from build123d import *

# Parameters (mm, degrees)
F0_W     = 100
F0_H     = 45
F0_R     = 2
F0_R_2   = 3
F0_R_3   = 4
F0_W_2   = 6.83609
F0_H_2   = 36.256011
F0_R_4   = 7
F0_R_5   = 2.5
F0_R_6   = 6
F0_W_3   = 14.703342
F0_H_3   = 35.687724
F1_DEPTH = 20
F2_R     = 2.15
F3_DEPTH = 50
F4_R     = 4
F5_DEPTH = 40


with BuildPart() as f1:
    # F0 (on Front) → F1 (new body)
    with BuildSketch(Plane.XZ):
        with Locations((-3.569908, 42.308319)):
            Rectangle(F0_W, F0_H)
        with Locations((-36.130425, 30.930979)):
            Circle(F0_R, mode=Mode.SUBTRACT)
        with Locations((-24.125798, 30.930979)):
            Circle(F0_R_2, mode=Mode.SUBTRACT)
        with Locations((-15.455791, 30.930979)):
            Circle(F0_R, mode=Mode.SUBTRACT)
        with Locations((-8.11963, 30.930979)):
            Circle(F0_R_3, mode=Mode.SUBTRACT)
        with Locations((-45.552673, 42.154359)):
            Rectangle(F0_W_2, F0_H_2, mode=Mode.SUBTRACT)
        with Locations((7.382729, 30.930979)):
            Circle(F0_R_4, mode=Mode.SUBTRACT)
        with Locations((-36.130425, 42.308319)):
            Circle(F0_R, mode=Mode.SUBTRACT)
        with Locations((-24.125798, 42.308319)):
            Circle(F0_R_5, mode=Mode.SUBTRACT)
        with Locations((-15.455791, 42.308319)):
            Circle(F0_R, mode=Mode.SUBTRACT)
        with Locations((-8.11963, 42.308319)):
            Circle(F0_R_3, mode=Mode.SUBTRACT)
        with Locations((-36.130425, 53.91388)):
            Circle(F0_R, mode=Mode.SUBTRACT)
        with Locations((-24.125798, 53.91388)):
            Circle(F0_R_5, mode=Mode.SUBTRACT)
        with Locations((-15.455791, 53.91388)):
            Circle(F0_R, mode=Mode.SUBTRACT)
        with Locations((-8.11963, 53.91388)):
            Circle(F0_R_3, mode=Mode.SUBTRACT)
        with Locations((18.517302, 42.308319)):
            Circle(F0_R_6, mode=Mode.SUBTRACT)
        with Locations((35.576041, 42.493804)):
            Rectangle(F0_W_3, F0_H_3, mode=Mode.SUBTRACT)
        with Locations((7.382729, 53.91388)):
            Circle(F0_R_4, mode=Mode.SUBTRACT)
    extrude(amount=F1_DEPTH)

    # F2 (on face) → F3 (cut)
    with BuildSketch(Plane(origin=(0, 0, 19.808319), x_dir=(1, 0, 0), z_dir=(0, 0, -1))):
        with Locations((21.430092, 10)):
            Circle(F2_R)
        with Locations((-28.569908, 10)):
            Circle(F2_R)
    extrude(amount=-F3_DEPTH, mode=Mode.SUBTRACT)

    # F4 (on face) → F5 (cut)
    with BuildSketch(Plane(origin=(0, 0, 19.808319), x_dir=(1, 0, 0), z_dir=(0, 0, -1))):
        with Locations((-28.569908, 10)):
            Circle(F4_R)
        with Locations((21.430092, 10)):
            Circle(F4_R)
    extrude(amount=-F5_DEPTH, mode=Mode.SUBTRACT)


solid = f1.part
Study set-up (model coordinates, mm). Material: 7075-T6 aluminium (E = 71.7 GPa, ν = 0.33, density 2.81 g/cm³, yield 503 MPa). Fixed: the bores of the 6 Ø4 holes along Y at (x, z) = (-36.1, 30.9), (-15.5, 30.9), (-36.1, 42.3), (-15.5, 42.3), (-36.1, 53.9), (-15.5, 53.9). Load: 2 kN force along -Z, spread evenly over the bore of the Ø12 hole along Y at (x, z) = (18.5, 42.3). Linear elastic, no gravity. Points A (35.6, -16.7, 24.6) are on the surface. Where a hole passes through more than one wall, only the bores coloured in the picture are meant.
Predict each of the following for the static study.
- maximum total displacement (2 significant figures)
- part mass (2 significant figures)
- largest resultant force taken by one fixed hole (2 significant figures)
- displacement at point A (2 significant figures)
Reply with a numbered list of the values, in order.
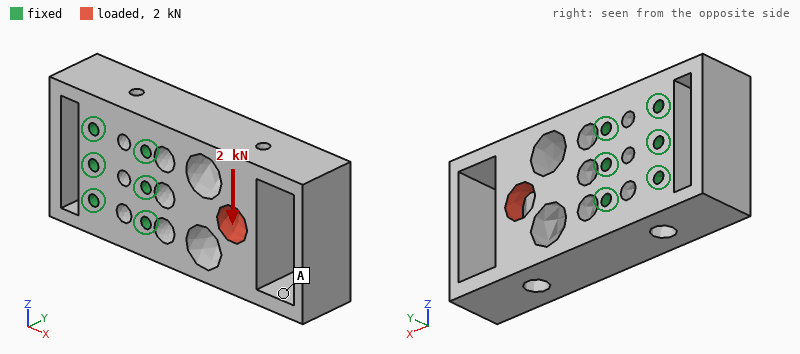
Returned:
1. 24 µm
2. 160 g
3. 1.9 kN
4. 21 µm
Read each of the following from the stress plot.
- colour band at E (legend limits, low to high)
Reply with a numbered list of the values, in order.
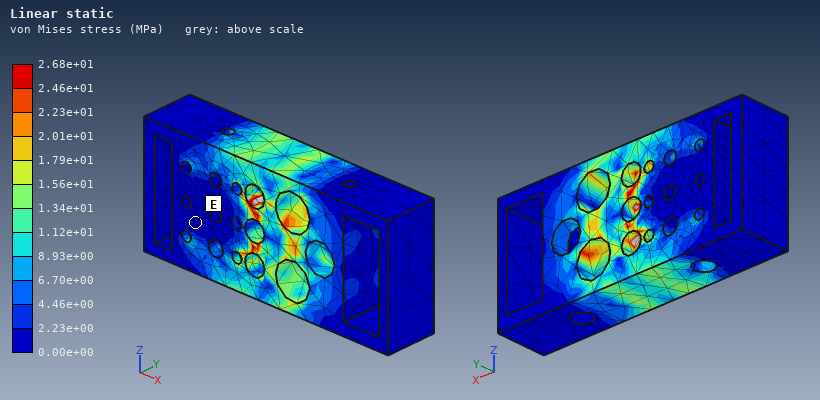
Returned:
1. 0.00e+00 to 2.23e+00 MPa
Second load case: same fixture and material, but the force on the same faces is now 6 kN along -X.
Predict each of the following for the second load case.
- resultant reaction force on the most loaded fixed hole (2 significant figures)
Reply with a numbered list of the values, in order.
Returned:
1. 2.0 kN
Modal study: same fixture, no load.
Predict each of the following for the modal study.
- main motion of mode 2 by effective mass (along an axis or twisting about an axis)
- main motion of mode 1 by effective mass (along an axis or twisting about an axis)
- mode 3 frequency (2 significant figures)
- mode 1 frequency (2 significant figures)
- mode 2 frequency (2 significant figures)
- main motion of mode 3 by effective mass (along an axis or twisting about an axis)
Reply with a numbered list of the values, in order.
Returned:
1. along Z
2. along Y
3. 6800 Hz
4. 3700 Hz
5. 4900 Hz
6. twisting about X
